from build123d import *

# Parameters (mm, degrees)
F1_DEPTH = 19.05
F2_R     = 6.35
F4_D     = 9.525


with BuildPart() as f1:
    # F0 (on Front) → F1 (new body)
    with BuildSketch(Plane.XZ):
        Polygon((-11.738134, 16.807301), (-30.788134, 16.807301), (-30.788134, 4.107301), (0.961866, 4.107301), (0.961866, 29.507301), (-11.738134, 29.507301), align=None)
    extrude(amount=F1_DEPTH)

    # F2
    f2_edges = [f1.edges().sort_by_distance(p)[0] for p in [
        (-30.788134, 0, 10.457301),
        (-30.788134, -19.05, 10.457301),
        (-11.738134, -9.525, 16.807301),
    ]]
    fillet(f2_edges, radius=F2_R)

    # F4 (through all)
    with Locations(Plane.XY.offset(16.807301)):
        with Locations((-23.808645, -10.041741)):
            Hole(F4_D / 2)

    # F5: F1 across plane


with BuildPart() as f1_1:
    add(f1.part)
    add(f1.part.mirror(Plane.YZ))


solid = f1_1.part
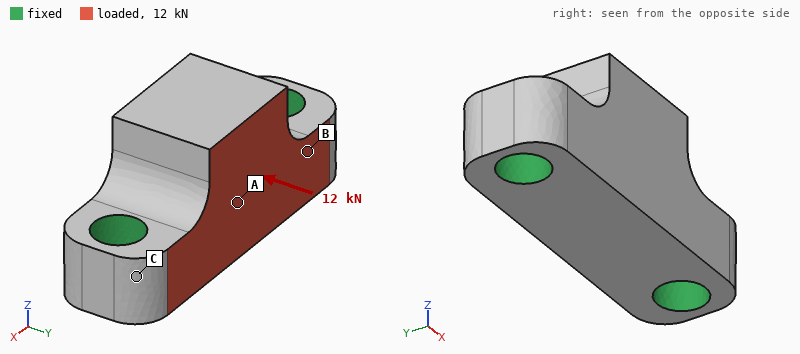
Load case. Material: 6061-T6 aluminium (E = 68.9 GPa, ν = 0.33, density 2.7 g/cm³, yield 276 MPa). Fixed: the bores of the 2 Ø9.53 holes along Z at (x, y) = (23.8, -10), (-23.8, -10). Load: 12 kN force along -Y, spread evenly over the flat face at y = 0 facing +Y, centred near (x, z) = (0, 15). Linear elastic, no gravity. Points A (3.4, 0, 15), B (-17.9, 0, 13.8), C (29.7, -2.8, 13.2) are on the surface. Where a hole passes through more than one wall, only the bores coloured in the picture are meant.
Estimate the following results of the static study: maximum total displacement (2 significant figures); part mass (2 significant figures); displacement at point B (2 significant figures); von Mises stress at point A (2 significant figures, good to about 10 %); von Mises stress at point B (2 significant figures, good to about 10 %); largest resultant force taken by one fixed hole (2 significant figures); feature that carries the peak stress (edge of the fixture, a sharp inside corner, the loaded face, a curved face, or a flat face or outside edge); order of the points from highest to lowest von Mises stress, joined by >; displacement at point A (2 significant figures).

46 µm
50 g
10 µm
34 MPa
54 MPa
6.1 kN
edge of the fixture
B > A > C
25 µm
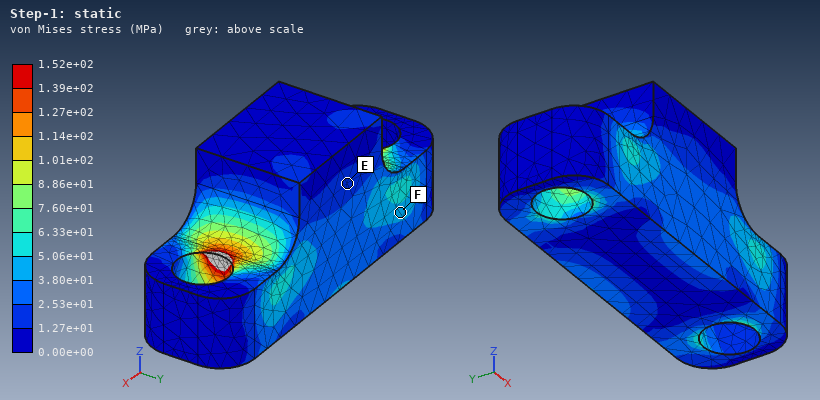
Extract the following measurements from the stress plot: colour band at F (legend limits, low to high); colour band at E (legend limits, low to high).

3.80e+01 to 5.06e+01 MPa
1.27e+01 to 2.53e+01 MPa
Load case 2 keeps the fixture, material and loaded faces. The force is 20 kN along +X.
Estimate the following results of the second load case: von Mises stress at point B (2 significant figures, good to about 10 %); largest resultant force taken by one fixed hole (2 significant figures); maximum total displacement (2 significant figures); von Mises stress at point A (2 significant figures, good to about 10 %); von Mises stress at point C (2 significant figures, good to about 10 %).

44 MPa
11 kN
31 µm
52 MPa
14 MPa
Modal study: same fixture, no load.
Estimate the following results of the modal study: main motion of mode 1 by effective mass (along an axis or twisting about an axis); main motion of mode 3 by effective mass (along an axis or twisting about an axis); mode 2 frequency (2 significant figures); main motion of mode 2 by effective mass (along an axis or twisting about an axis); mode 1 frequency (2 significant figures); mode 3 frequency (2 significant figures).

along Y
along Y
23 kHz
along Z
14 kHz
27 kHz
